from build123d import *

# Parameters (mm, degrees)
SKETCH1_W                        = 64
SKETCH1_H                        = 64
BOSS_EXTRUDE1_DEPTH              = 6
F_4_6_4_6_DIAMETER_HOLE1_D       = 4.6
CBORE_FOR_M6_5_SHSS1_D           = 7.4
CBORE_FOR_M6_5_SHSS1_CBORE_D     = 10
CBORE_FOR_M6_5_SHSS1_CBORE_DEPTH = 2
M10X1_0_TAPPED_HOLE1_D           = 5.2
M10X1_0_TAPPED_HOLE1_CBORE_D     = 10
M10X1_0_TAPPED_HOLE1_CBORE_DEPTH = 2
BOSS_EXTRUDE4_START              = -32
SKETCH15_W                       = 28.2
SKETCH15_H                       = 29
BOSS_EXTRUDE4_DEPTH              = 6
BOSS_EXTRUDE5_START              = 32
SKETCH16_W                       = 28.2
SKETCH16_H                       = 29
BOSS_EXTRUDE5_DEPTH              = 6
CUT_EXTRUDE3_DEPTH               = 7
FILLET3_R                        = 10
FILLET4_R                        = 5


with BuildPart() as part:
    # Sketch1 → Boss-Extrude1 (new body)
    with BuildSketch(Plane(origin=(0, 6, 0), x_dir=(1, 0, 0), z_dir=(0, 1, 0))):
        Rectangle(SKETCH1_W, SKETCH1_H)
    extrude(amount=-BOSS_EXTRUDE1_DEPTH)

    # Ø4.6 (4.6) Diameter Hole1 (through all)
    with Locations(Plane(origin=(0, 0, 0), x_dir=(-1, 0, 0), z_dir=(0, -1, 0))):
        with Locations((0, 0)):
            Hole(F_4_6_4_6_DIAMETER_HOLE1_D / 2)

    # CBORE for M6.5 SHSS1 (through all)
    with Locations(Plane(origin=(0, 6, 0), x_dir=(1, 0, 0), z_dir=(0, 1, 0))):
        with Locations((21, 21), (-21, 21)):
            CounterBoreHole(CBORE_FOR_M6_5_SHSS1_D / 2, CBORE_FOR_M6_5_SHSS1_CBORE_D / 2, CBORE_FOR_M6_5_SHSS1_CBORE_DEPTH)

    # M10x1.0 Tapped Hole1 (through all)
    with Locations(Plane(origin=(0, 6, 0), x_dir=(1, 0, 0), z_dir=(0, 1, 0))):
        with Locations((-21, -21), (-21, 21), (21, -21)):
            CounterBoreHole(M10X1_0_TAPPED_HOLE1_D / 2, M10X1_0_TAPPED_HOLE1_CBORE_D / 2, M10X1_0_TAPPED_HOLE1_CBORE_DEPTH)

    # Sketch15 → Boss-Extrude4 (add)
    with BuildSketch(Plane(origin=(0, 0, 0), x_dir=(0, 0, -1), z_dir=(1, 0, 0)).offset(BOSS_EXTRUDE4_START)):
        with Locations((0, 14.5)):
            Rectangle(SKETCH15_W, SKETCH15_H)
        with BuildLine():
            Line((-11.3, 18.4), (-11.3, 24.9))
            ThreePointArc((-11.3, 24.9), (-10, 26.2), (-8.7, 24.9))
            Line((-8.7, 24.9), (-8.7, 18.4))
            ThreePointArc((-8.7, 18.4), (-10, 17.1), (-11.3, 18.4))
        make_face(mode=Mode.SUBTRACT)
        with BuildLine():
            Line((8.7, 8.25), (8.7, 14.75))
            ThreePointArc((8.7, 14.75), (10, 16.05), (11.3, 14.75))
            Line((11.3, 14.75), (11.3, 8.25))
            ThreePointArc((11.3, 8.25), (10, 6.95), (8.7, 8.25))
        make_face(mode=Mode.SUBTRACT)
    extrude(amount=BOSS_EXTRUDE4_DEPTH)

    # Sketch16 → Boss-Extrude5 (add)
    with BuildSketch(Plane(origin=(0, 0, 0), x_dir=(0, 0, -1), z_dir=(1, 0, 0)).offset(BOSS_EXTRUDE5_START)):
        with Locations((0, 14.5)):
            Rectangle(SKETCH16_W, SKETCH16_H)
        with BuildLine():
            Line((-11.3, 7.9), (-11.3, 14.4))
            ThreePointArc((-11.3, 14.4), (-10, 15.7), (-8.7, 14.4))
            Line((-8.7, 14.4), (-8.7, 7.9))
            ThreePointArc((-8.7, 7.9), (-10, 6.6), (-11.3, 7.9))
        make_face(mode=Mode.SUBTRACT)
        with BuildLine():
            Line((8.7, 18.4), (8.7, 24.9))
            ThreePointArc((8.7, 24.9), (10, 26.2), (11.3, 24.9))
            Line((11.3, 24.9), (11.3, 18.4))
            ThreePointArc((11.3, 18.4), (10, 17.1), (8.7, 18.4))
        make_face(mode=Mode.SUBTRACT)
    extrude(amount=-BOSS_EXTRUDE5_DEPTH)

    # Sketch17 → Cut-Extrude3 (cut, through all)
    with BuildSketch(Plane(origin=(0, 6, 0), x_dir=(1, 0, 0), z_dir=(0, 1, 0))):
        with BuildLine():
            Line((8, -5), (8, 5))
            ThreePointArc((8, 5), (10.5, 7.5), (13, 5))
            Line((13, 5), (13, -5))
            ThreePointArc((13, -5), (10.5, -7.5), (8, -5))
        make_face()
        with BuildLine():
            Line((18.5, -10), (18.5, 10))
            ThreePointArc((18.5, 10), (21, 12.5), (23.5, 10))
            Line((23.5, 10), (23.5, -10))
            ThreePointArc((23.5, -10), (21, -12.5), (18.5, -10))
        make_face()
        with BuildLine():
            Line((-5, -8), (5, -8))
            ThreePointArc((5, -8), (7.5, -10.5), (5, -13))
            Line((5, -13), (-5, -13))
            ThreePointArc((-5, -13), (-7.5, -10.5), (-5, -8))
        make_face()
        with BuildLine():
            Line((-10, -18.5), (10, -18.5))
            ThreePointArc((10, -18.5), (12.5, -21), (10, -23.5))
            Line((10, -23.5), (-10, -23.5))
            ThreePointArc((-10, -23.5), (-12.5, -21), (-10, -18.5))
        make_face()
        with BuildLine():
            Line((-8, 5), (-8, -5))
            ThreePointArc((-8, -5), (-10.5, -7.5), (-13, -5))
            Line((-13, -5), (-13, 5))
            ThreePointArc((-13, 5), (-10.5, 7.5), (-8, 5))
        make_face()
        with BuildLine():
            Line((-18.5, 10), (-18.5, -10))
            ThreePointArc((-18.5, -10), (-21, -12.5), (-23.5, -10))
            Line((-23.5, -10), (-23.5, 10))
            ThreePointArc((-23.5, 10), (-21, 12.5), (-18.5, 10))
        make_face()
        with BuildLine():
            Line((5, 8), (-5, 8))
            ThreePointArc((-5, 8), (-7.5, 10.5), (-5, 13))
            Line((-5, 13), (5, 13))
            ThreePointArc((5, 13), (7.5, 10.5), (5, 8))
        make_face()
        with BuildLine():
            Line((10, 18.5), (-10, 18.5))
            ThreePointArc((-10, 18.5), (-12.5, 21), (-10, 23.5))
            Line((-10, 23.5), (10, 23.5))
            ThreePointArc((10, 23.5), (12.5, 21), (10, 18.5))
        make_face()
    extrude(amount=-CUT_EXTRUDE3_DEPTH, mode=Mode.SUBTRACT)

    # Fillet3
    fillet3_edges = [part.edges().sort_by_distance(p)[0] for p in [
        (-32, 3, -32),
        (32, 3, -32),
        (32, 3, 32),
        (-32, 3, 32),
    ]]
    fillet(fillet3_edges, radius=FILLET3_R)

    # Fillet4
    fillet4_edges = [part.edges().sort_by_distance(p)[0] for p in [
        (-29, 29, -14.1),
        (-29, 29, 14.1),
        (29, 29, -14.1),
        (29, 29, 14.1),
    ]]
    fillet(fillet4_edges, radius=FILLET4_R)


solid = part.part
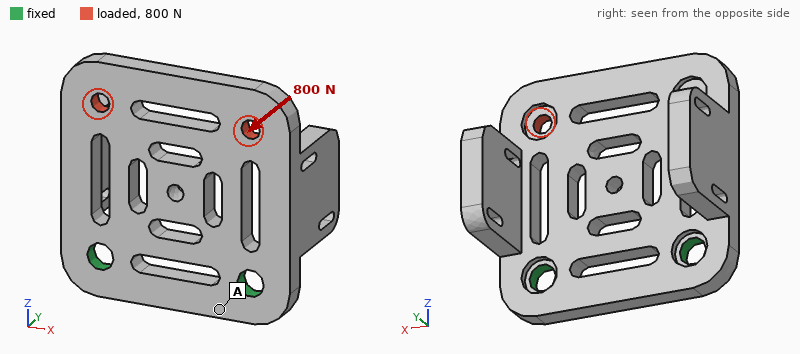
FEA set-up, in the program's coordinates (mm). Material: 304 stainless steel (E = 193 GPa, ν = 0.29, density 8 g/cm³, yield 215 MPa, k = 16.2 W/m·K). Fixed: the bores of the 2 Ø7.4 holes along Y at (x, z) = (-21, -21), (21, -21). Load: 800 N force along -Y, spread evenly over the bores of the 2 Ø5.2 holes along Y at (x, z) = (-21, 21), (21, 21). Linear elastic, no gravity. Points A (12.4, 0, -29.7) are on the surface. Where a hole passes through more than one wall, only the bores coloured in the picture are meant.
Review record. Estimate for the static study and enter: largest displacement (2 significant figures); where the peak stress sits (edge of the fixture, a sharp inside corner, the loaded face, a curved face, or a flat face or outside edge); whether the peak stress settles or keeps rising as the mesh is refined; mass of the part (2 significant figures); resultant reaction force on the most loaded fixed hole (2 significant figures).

0.17 mm
edge of the fixture
keeps rising
200 g
400 N
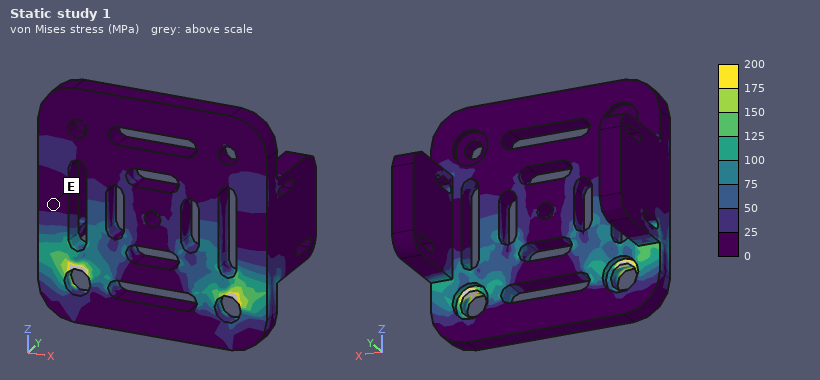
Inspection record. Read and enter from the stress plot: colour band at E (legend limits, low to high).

0 to 25 MPa
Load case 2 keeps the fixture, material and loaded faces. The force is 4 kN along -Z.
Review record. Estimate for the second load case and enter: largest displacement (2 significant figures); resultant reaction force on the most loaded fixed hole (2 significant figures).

28 µm
2.0 kN
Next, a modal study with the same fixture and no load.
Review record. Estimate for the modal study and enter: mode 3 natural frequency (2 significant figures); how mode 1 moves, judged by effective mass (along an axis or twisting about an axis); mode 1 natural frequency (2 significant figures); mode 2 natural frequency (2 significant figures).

3400 Hz
along Y
1400 Hz
2200 Hz
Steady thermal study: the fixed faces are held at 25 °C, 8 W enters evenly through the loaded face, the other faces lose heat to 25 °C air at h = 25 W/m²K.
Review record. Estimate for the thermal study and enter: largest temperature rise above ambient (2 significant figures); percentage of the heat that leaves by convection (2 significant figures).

48 K
67 %
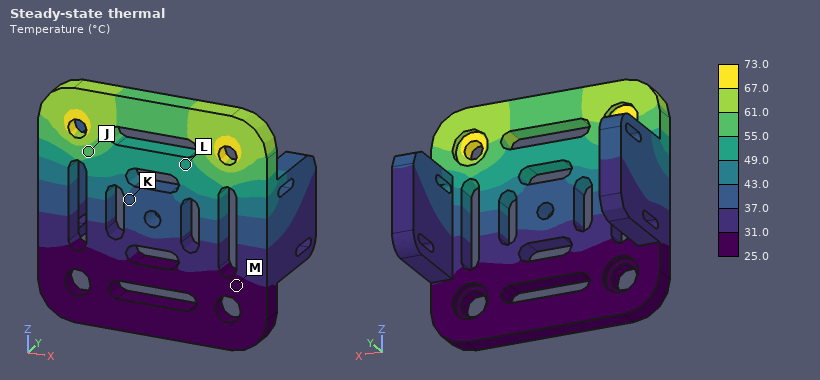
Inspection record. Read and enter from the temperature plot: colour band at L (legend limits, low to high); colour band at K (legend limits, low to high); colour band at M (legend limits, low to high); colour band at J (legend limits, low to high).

49.0 to 55.0 °C
37.0 to 43.0 °C
25.0 to 31.0 °C
55.0 to 61.0 °C
